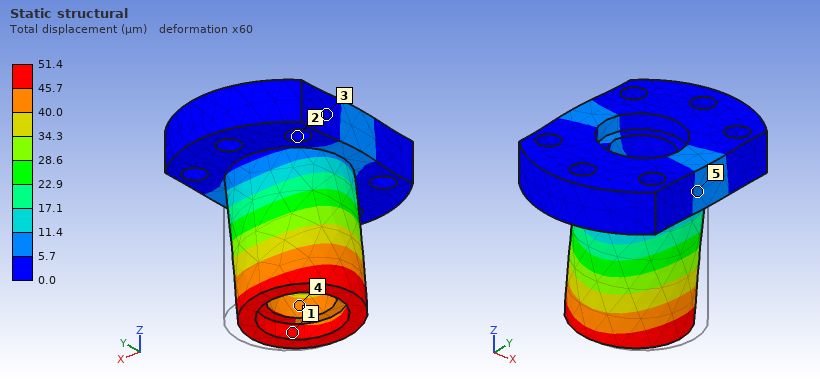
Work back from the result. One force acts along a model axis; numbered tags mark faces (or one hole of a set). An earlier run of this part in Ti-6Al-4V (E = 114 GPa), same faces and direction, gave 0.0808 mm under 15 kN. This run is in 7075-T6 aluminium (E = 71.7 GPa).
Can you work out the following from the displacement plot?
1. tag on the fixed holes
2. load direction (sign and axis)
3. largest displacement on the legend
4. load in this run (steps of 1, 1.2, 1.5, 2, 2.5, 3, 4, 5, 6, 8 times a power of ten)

2
-X
51.4 µm
6 kN
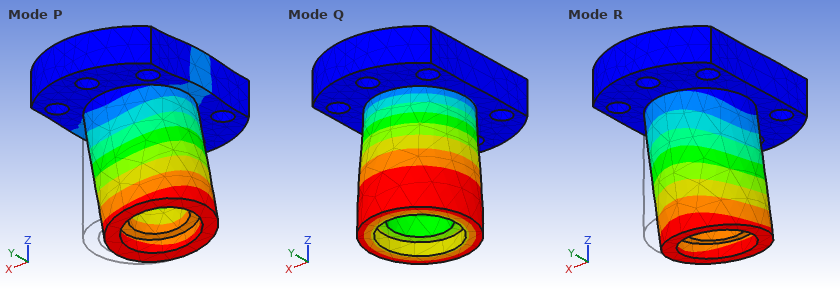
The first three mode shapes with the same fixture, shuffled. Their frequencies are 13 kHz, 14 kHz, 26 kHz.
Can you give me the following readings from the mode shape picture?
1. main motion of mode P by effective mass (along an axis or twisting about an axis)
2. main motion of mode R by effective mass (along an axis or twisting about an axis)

along X
along Y
